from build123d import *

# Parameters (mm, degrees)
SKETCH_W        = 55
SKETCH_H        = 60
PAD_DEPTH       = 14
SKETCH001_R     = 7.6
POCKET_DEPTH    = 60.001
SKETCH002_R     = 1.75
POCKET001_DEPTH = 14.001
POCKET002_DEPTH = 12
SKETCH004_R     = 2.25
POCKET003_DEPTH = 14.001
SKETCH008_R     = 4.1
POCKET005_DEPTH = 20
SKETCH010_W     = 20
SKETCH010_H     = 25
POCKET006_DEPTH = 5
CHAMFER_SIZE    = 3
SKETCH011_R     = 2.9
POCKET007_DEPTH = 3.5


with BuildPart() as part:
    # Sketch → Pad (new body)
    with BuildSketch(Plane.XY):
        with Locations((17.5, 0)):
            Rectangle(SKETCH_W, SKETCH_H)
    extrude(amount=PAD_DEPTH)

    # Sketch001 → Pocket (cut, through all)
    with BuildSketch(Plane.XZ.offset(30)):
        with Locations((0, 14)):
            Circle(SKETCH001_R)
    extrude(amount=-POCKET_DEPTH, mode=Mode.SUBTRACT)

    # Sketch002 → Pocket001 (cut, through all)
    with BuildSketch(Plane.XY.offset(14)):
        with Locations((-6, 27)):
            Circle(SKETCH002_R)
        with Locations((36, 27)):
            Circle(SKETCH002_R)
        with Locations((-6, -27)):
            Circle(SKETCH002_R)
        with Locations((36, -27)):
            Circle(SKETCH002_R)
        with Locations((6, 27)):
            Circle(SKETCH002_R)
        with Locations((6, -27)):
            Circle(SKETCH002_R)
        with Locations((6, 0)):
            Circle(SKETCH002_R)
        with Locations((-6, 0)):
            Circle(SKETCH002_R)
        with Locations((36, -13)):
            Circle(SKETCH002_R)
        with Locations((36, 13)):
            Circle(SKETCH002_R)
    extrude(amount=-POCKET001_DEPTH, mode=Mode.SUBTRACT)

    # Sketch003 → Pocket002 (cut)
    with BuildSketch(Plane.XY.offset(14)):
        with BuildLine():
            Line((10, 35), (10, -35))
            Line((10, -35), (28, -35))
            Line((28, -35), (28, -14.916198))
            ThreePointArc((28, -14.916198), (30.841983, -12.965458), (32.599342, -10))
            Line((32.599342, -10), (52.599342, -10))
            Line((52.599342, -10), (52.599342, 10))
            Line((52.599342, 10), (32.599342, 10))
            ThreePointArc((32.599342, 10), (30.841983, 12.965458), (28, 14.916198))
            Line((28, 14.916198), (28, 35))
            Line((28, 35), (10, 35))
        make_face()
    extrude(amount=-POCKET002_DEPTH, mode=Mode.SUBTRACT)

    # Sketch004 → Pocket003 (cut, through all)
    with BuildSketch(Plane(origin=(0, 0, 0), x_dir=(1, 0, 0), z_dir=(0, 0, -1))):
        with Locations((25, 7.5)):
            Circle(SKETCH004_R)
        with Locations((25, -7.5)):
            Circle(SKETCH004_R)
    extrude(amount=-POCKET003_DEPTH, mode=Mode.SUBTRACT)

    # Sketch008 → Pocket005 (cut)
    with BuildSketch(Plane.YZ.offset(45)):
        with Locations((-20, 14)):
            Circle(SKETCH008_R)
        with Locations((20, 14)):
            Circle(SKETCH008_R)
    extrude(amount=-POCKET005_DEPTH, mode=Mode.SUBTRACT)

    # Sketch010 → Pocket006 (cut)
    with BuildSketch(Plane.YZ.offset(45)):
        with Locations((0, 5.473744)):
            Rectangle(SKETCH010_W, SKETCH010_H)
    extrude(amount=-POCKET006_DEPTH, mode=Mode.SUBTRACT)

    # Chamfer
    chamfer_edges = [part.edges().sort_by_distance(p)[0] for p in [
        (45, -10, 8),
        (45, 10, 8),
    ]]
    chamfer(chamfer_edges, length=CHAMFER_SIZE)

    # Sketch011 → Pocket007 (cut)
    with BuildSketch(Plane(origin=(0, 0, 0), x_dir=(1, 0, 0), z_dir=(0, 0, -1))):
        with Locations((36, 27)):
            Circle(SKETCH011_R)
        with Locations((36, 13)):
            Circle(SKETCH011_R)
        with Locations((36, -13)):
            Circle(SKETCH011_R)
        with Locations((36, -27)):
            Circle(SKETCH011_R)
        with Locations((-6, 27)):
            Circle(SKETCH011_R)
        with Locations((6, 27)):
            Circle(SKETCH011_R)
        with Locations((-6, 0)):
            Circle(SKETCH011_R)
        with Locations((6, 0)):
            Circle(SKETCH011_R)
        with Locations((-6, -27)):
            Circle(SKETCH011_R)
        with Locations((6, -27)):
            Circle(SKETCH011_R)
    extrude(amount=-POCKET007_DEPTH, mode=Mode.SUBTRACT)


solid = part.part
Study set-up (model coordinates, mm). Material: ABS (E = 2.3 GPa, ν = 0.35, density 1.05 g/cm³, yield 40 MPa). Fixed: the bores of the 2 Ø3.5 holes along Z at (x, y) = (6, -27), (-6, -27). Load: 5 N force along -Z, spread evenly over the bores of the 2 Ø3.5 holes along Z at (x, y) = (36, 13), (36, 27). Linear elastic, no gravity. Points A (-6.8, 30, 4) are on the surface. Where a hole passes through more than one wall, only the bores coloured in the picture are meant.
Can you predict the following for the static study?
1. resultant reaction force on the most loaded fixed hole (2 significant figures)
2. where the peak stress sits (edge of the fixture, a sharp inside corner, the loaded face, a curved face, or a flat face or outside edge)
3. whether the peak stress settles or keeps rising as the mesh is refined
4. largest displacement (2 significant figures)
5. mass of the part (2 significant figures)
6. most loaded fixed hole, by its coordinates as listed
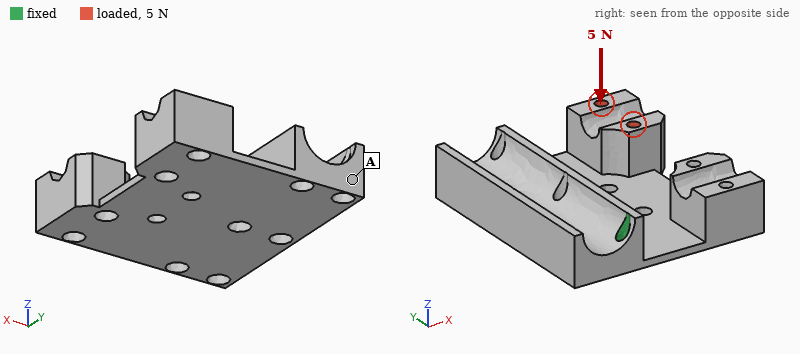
13 N
edge of the fixture
keeps rising
0.97 mm
21 g
(6, -27)
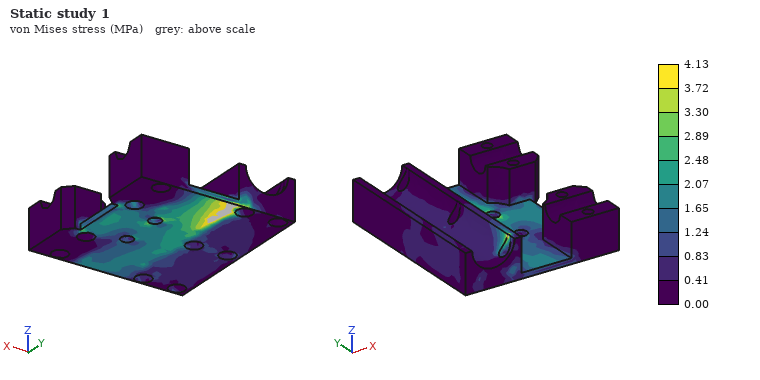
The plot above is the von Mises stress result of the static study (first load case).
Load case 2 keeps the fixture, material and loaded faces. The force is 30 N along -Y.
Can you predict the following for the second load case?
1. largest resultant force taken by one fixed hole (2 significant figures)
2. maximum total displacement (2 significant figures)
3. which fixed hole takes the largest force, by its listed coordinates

87 N
0.97 mm
(6, -27)
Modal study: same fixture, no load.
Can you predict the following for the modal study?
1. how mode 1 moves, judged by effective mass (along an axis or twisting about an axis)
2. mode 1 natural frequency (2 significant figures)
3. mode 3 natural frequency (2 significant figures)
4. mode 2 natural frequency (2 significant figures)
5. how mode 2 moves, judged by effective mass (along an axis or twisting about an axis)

along Z
180 Hz
660 Hz
280 Hz
twisting about X
